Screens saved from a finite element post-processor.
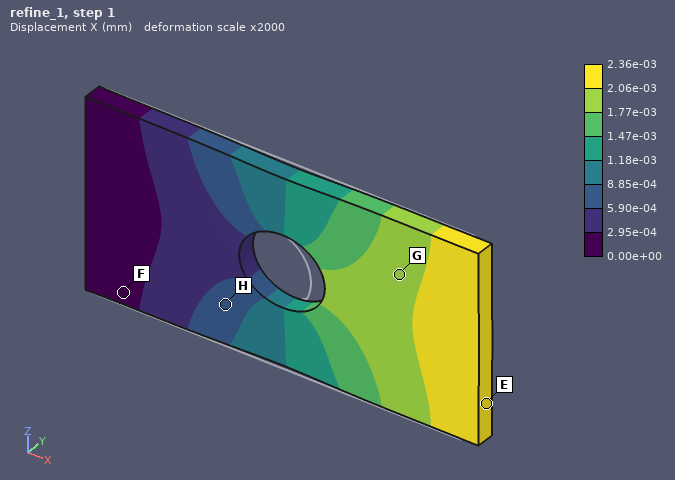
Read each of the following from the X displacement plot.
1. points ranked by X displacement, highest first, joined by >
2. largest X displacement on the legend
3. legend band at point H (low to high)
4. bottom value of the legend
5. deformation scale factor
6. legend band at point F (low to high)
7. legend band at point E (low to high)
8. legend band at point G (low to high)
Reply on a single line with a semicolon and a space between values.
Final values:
E > G > H > F; 2.36e-03 mm; 5.90e-04 to 8.85e-04 mm; 0.00e+00 mm; 2000; 0.00e+00 to 2.95e-04 mm; 2.06e-03 to 2.36e-03 mm; 1.77e-03 to 2.06e-03 mm
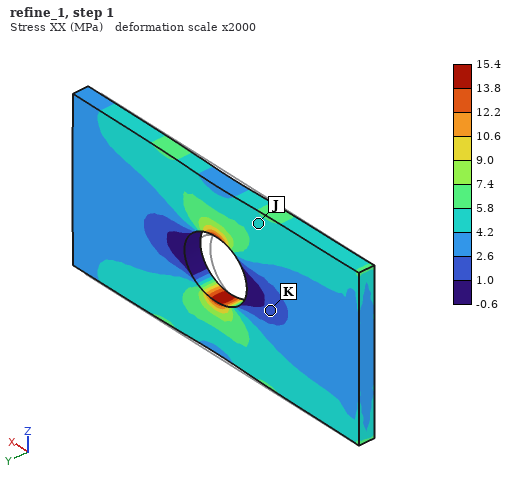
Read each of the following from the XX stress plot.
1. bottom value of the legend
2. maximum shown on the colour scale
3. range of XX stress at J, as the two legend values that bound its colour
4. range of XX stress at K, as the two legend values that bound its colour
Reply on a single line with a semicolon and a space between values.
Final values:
-0.6 MPa; 15.4 MPa; 4.2 to 5.8 MPa; 1.0 to 2.6 MPa
